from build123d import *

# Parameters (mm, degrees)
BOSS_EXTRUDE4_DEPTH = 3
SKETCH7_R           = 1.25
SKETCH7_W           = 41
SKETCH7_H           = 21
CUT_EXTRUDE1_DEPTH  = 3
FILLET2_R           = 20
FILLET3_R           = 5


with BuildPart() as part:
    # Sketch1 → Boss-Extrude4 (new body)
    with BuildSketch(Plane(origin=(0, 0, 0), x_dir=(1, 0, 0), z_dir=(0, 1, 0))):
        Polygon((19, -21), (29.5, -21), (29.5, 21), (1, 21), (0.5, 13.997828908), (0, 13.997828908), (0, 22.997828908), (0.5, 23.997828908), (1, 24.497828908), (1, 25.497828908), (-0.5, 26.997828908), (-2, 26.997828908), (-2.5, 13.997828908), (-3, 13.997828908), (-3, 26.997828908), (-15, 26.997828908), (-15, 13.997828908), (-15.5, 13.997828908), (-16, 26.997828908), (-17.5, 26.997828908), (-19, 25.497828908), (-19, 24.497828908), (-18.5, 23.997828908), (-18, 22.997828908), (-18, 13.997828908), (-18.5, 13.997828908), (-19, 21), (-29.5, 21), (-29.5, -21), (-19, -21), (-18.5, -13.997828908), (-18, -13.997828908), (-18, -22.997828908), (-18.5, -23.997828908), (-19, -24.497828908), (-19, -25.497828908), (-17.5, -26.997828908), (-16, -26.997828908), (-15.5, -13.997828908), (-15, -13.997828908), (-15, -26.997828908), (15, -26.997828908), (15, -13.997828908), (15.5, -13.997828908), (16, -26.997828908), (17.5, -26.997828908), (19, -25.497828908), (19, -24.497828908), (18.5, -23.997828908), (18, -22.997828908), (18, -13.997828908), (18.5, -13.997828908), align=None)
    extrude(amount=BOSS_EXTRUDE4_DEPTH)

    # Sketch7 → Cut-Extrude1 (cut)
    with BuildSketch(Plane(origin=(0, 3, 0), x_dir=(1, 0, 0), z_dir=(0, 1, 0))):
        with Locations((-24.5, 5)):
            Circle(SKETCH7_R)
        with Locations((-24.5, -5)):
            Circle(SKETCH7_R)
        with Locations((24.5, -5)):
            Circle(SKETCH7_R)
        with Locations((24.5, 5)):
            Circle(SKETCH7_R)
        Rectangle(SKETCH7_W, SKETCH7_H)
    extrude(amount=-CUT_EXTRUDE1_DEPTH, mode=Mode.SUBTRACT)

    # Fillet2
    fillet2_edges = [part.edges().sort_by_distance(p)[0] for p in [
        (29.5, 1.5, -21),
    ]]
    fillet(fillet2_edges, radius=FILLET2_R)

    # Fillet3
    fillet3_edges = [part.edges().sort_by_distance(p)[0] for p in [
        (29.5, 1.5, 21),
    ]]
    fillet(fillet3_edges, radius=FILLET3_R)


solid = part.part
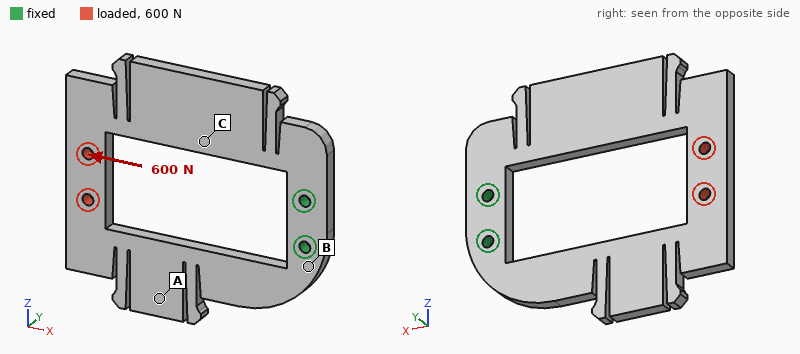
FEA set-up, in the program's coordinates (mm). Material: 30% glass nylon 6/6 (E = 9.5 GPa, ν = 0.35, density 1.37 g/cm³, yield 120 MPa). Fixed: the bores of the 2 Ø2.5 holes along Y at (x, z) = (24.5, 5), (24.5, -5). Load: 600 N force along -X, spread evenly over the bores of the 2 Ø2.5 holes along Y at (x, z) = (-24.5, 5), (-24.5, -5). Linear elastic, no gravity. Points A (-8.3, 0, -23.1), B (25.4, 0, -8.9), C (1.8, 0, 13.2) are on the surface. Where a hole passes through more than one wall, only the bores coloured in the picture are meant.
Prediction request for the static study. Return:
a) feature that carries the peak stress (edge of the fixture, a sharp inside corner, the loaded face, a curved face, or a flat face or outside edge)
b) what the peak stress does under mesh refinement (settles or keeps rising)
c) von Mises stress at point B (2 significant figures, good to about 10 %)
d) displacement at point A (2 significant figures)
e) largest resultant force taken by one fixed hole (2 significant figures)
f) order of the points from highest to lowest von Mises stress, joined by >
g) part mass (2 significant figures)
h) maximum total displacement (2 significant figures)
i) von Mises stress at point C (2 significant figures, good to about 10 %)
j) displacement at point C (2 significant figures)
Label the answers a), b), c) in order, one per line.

a) edge of the fixture
b) keeps rising
c) 30 MPa
d) 0.23 mm
e) 310 N
f) B > C > A
g) 7.3 g
h) 0.31 mm
i) 16 MPa
j) 0.15 mm
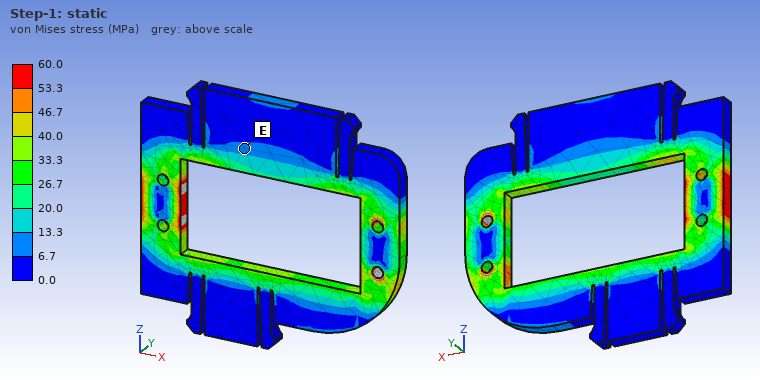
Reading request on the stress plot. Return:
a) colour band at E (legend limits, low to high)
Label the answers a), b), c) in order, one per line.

a) 6.7 to 13.3 MPa
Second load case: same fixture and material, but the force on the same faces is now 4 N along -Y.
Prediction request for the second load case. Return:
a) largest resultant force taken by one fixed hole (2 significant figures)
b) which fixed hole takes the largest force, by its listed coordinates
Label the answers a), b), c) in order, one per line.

a) 2.4 N
b) (24.5, -5)
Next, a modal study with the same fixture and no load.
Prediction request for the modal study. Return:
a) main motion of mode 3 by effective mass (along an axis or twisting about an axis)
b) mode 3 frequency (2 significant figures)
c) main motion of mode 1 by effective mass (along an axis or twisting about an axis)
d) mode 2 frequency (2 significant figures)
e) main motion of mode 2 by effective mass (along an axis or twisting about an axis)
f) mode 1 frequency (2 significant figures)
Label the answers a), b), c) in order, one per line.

a) along Z
b) 600 Hz
c) along Y
d) 480 Hz
e) twisting about X
f) 240 Hz
